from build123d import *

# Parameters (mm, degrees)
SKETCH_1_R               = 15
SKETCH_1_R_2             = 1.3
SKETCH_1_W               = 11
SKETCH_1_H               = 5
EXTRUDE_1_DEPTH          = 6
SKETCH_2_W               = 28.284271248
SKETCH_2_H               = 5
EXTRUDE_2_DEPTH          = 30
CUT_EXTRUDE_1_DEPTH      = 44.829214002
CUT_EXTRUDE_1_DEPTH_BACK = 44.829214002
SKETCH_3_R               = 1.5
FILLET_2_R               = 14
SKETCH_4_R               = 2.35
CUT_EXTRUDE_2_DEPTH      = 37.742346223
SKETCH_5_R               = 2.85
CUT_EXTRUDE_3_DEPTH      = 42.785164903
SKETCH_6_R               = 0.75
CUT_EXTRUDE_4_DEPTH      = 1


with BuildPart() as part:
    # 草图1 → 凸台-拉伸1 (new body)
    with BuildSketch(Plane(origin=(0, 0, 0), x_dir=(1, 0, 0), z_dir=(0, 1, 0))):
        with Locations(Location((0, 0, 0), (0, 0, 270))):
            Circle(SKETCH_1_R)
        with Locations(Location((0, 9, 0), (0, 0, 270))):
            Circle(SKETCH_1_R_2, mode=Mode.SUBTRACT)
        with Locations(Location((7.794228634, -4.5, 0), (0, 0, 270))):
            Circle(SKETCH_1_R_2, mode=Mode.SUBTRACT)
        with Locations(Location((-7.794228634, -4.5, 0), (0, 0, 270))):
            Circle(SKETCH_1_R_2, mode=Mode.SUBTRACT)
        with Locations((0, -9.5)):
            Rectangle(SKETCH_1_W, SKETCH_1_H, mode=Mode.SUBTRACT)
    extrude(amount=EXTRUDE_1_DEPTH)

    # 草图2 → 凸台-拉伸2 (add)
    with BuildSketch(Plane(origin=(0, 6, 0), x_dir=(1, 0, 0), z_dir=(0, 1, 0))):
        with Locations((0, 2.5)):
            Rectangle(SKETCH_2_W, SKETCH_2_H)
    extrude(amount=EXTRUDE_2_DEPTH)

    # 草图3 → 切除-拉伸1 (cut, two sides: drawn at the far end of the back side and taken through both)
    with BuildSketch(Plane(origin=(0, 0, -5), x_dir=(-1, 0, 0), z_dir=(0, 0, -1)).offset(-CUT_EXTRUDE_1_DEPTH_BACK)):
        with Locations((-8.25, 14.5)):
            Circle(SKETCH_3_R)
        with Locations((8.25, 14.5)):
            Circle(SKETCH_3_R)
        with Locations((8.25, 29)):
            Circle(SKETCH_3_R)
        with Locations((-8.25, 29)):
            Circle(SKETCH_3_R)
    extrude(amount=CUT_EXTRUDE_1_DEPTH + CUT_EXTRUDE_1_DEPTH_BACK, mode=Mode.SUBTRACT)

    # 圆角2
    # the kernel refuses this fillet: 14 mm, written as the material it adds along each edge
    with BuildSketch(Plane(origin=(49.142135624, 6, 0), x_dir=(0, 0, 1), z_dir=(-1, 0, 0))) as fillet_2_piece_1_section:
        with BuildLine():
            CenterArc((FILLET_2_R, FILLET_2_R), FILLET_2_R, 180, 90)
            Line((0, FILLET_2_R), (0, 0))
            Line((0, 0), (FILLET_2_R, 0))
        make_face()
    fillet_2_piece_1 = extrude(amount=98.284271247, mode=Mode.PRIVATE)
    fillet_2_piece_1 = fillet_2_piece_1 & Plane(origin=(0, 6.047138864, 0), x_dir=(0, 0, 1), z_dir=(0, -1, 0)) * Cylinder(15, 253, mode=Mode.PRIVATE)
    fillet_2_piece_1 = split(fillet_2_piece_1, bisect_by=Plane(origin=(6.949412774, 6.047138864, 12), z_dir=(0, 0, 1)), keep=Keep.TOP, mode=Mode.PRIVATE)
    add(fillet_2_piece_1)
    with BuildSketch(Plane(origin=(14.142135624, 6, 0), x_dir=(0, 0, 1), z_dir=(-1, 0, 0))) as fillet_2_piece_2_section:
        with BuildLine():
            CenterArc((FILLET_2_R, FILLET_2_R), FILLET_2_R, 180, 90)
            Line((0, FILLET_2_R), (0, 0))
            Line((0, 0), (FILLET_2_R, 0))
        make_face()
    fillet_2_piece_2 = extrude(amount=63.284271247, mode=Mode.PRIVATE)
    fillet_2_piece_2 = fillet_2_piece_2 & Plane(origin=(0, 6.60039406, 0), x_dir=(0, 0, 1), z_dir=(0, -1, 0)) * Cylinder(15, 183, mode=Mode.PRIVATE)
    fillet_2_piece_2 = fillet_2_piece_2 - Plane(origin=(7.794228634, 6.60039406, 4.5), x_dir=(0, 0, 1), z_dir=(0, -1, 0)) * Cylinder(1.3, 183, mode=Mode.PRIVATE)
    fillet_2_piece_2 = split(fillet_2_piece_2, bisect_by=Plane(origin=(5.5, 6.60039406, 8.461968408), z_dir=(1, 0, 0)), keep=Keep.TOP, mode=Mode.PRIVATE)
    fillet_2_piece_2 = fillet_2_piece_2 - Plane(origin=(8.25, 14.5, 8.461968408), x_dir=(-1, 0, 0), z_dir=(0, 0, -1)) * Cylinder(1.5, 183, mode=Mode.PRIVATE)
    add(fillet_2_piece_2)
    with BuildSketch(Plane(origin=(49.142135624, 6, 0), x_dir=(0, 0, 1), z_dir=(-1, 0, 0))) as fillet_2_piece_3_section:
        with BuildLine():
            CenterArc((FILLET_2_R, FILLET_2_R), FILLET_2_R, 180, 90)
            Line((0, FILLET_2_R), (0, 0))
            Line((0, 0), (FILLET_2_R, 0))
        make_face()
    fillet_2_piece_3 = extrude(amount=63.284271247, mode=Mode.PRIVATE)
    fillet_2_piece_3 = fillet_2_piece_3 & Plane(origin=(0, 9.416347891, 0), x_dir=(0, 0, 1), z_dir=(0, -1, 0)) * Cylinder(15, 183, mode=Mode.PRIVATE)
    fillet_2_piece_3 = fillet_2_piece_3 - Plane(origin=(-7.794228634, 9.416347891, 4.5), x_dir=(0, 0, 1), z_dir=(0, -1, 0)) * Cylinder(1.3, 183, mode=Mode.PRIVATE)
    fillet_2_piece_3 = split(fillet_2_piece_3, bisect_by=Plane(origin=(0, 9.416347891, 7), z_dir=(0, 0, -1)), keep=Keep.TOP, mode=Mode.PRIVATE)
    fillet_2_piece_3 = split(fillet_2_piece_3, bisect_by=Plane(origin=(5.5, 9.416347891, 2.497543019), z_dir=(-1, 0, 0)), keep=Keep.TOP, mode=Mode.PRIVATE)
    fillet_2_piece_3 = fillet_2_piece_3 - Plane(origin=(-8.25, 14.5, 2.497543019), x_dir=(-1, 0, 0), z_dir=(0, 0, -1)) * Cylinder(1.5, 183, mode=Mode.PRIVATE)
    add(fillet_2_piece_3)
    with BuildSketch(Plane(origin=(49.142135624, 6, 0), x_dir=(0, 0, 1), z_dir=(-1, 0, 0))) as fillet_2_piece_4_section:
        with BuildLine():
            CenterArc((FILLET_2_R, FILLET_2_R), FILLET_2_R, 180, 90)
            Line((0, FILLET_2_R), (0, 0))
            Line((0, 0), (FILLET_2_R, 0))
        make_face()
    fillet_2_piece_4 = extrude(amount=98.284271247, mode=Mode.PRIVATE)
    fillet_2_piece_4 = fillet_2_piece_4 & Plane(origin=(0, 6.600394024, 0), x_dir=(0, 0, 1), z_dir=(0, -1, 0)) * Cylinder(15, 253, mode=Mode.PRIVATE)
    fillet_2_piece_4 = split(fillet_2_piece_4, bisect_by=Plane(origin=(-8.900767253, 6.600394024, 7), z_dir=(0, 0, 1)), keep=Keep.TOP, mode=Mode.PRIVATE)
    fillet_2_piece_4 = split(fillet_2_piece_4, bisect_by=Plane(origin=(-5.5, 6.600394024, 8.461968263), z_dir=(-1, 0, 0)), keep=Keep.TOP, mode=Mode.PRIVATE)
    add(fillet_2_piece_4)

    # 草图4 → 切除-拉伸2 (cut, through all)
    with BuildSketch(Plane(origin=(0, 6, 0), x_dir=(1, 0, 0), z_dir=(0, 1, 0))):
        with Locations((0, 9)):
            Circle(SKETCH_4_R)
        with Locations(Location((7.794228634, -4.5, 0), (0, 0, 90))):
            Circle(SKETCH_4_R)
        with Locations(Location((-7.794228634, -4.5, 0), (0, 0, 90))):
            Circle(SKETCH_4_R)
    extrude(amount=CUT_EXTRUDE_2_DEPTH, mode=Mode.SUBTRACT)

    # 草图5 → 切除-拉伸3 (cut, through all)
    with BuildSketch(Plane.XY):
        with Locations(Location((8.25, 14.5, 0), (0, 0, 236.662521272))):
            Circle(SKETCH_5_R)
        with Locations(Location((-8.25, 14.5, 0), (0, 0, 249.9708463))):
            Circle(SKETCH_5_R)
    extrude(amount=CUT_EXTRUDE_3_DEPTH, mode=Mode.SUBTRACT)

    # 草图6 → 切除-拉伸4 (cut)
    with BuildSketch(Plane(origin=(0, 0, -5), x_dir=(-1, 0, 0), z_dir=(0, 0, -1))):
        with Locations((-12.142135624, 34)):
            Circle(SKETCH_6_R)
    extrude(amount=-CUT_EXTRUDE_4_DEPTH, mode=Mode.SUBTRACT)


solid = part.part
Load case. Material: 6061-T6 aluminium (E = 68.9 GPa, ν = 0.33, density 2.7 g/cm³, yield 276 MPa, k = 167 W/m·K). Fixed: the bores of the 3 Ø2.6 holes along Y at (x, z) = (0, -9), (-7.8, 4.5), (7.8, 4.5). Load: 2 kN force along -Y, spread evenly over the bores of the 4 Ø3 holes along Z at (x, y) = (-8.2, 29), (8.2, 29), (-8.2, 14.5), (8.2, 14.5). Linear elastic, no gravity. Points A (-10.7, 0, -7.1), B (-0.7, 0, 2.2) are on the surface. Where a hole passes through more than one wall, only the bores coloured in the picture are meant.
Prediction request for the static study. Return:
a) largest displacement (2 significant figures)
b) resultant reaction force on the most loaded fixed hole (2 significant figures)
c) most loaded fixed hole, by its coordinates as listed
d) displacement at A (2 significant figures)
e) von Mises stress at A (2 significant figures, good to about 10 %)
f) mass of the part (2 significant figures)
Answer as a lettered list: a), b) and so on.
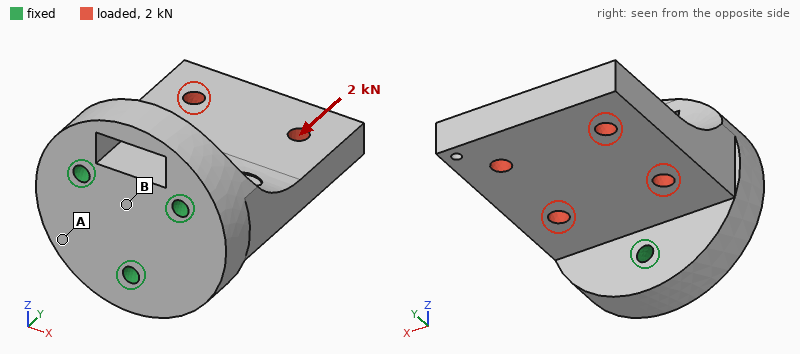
a) 19 µm
b) 890 N
c) (0, -9)
d) 4.0 µm
e) 11 MPa
f) 24 g
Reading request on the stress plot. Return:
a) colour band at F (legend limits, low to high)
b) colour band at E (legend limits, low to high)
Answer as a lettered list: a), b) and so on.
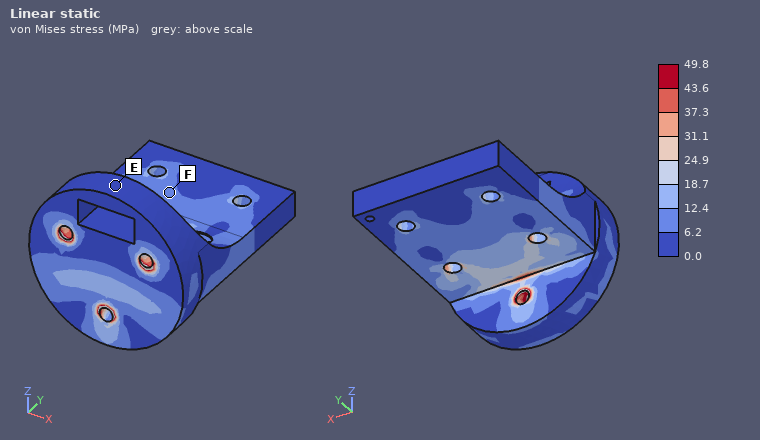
a) 6.2 to 12.4 MPa
b) 0.0 to 6.2 MPa
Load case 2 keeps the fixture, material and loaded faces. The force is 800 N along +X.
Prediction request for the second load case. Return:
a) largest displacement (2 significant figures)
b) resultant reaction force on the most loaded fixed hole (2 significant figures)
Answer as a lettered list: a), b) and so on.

a) 19 µm
b) 790 N
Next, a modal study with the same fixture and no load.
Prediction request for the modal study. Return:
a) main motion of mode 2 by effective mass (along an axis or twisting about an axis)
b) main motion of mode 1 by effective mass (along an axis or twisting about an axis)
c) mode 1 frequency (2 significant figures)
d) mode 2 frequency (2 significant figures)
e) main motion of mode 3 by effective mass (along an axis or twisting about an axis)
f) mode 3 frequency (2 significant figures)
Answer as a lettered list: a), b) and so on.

a) along X
b) along Z
c) 6000 Hz
d) 11 kHz
e) along X
f) 13 kHz
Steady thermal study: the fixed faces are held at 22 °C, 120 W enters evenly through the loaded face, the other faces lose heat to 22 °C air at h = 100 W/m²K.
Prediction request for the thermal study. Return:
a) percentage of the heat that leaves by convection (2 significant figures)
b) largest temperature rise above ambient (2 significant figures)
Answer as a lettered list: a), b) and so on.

a) 11 %
b) 82 K
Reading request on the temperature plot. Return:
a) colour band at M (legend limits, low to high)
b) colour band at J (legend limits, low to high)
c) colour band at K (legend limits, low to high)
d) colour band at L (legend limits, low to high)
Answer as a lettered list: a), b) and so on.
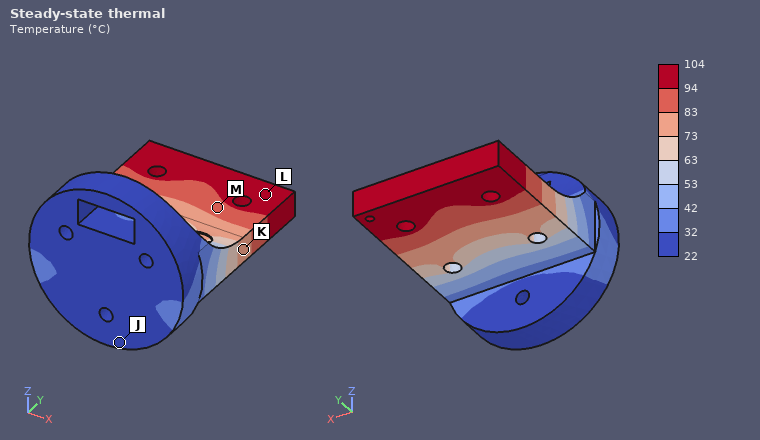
a) 83 to 94 °C
b) 22 to 32 °C
c) 73 to 83 °C
d) 94 to 104 °C
